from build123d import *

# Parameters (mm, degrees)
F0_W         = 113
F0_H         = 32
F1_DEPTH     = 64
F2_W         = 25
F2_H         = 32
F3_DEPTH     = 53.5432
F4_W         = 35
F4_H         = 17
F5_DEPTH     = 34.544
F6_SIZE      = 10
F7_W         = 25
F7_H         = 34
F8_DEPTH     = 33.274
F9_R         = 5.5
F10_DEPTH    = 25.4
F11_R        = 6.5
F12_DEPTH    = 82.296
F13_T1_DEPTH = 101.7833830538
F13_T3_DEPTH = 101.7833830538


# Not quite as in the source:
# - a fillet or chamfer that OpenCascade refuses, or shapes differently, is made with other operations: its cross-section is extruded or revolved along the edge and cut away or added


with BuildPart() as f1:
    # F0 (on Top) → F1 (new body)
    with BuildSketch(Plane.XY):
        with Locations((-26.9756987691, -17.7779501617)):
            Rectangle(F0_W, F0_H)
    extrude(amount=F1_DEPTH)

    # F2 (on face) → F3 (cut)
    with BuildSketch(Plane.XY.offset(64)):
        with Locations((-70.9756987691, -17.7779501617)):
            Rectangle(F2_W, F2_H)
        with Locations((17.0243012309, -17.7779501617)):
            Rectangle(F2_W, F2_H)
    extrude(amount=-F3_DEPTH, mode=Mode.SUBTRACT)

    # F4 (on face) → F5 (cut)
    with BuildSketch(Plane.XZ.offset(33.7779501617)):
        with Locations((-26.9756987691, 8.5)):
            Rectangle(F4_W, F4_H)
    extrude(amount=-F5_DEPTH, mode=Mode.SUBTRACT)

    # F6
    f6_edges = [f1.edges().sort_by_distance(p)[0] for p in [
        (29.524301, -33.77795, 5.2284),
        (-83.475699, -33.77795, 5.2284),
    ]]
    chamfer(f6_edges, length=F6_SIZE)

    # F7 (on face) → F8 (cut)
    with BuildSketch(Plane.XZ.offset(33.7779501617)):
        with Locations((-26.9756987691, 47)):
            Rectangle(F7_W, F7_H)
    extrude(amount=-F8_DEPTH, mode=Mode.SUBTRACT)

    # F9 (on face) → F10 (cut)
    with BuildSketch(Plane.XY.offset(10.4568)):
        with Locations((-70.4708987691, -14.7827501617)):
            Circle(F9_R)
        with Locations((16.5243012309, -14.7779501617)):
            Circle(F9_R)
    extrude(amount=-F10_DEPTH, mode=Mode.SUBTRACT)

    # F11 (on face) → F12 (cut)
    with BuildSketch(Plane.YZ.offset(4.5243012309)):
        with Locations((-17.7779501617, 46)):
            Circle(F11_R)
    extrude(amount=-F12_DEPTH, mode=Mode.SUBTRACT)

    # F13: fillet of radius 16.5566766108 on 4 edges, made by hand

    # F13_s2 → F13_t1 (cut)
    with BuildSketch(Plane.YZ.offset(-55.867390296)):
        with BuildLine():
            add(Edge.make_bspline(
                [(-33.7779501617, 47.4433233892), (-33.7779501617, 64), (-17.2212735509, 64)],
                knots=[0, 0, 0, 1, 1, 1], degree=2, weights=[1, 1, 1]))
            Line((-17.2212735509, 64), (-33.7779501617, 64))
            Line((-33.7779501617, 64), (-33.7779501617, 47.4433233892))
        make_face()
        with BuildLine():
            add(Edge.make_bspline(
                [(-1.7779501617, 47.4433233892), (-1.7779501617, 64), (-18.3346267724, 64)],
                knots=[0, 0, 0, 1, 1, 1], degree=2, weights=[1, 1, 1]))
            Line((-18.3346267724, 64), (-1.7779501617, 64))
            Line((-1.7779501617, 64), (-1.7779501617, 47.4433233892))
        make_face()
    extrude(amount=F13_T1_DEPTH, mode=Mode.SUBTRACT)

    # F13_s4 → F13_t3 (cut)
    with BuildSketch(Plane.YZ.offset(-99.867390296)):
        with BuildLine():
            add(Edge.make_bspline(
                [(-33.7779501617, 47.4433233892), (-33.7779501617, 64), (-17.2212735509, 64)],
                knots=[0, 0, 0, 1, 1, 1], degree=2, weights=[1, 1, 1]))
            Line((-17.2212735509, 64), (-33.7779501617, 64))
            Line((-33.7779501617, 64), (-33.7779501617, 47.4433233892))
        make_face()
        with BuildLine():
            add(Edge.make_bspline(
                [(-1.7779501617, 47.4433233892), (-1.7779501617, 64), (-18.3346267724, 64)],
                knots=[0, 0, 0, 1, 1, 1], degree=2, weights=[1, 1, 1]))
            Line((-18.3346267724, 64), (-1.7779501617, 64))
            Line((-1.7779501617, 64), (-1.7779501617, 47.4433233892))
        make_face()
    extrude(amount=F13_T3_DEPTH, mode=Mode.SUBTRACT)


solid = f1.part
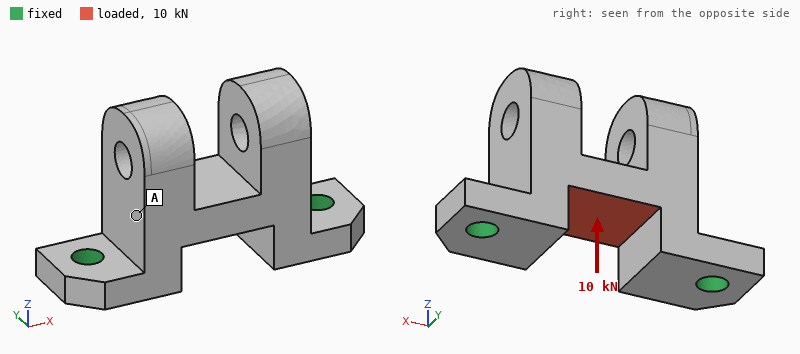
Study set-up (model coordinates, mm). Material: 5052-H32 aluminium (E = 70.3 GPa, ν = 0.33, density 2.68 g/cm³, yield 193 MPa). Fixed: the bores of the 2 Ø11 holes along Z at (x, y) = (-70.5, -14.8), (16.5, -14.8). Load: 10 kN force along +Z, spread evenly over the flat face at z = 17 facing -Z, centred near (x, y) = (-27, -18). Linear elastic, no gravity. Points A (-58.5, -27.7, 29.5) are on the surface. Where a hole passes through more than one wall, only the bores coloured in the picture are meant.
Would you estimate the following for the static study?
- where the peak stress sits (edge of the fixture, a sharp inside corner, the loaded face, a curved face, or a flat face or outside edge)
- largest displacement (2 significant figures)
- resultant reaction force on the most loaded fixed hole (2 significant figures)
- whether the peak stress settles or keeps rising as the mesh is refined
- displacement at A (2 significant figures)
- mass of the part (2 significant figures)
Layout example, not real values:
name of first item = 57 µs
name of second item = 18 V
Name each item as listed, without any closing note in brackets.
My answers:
where the peak stress sits = edge of the fixture
largest displacement = 54 µm
resultant reaction force on the most loaded fixed hole = 7.1 kN
whether the peak stress settles or keeps rising as the mesh is refined = keeps rising
displacement at A = 24 µm
mass of the part = 240 g
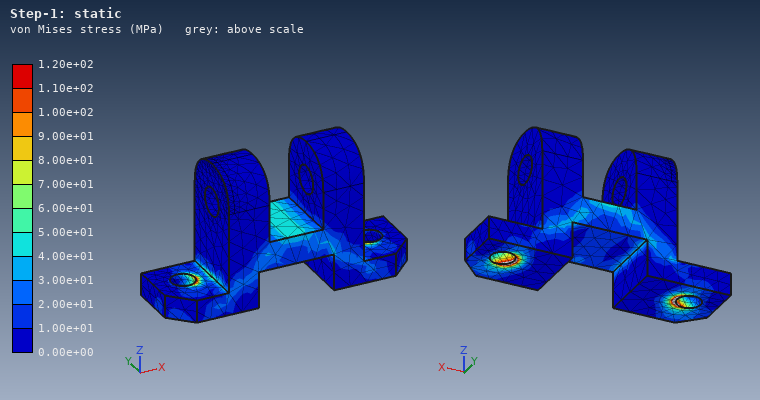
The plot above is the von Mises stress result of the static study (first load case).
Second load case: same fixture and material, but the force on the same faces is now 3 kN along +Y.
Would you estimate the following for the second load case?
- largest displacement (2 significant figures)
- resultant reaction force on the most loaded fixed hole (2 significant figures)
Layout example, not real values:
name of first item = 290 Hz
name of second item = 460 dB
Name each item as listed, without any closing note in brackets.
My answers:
largest displacement = 50 µm
resultant reaction force on the most loaded fixed hole = 1.5 kN
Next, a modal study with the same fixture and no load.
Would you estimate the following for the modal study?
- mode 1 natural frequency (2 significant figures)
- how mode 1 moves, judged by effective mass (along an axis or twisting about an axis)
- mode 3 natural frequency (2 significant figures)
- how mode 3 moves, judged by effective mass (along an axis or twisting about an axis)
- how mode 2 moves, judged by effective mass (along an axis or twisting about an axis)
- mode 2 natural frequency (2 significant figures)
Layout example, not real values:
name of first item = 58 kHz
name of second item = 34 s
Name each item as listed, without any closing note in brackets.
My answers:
mode 1 natural frequency = 2400 Hz
how mode 1 moves, judged by effective mass = along Y
mode 3 natural frequency = 5600 Hz
how mode 3 moves, judged by effective mass = along X
how mode 2 moves, judged by effective mass = twisting about Z
mode 2 natural frequency = 4500 Hz
